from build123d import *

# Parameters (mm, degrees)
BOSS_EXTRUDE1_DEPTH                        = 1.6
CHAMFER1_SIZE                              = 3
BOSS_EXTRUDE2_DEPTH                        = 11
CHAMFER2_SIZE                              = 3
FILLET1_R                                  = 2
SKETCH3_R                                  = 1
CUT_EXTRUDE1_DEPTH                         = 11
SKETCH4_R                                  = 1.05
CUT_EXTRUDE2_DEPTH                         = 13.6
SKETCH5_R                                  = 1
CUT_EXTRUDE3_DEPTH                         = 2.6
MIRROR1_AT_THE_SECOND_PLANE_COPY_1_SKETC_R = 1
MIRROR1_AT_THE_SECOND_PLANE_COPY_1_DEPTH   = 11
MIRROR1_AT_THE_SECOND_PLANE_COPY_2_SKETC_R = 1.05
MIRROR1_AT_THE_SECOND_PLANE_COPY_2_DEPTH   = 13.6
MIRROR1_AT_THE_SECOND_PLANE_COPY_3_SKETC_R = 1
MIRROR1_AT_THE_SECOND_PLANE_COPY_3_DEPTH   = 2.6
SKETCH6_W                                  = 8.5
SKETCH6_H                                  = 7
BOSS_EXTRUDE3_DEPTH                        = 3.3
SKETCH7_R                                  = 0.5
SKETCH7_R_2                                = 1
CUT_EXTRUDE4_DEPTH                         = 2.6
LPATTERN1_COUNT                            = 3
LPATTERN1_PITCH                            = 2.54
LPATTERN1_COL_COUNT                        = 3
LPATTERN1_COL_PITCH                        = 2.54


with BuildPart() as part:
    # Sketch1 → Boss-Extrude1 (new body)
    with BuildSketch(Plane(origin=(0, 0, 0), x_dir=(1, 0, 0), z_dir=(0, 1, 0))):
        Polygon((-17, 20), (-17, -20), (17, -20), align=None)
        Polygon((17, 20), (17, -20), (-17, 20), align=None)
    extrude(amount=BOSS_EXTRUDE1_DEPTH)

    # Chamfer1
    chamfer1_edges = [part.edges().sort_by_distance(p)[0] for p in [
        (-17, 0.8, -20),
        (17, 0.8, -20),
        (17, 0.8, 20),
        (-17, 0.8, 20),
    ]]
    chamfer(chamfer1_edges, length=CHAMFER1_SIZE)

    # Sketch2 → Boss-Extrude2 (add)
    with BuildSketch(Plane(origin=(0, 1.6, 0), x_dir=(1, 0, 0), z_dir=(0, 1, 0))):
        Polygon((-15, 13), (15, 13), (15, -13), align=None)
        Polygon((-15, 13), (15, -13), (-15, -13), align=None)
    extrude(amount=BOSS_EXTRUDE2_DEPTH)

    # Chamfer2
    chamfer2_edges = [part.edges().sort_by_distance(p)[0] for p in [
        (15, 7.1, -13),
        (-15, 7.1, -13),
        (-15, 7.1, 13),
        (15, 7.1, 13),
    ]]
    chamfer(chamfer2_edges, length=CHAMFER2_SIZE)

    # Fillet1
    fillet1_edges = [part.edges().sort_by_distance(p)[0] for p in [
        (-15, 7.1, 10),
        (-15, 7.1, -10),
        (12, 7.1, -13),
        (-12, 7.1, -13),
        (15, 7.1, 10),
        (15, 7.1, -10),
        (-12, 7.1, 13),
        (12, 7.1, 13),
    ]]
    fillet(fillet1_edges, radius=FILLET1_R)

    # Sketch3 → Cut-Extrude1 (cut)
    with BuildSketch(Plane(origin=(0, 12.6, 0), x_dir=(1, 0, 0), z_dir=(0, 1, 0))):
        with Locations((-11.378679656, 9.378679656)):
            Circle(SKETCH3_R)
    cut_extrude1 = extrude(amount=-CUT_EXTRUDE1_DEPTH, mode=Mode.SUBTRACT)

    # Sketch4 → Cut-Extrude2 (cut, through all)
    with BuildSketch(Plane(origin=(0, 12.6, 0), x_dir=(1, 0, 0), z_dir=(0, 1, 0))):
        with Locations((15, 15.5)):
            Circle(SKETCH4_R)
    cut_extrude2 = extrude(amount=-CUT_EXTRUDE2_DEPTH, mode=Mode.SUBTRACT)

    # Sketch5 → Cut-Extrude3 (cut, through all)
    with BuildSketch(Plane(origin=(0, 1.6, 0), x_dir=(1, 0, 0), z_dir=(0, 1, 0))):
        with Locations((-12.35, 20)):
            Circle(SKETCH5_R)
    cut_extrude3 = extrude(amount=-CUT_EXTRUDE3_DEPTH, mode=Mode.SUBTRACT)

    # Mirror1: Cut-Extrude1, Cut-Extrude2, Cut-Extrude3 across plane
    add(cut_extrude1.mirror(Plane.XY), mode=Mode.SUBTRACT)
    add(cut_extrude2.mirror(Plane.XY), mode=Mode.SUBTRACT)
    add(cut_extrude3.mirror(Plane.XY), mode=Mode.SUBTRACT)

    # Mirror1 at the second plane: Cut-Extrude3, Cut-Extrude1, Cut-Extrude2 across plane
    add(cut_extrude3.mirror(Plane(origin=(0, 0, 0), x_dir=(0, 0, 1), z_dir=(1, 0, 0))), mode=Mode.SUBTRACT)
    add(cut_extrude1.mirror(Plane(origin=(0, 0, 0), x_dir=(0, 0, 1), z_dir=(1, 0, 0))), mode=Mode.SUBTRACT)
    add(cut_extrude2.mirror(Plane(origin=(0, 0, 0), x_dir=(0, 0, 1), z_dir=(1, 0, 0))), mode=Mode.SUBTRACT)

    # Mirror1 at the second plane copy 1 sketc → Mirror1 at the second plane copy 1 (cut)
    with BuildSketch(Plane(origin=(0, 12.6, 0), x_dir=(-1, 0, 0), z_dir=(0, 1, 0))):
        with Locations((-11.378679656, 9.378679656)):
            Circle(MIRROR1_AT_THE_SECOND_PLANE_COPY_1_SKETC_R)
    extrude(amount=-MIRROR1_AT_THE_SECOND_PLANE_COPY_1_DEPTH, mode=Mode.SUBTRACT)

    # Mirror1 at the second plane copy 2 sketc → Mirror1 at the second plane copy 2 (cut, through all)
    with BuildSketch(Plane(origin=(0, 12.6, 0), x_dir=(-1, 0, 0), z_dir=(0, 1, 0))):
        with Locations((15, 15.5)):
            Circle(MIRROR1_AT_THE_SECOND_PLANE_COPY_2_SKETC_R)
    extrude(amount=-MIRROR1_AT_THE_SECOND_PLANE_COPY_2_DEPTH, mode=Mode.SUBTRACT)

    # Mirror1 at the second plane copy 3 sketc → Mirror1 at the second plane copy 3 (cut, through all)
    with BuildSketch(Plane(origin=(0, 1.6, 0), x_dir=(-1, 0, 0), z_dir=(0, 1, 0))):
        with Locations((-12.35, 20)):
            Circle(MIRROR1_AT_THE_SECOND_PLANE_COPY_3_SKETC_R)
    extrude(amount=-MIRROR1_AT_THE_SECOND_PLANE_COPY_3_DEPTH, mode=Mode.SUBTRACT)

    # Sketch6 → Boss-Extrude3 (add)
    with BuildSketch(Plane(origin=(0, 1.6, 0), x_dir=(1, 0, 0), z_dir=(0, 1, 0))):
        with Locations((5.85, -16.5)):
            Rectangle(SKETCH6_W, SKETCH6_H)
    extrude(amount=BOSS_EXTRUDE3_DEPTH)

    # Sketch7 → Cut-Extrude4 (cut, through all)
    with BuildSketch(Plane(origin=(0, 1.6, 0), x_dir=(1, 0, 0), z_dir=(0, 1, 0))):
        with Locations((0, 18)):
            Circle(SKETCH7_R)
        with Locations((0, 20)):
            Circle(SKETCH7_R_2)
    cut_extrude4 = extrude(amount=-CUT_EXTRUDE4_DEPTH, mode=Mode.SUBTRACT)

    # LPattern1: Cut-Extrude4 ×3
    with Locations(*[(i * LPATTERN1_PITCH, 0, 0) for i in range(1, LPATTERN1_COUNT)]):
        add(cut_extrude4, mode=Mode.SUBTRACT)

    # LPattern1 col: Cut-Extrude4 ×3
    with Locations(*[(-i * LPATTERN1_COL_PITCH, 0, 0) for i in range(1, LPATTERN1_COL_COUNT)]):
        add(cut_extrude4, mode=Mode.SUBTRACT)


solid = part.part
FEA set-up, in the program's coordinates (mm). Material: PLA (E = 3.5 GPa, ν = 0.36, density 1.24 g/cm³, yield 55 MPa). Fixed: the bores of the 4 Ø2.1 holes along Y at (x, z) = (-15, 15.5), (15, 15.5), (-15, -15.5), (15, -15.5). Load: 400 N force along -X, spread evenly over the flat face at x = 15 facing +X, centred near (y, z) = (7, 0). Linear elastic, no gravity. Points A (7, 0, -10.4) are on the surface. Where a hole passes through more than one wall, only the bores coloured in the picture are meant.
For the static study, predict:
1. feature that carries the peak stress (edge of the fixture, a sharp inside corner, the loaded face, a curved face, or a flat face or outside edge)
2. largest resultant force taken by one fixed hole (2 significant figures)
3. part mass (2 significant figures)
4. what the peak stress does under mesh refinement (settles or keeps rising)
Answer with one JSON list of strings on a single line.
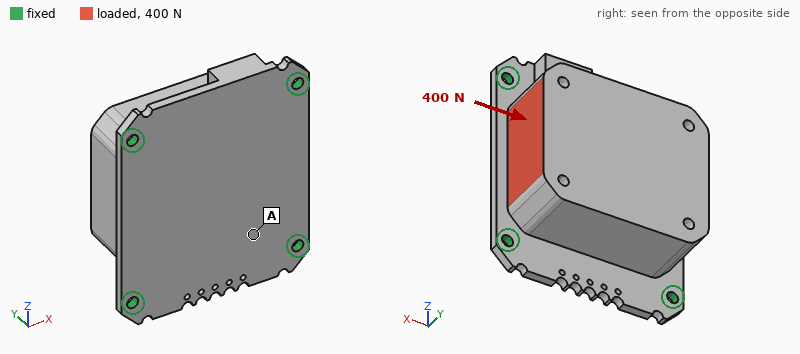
["edge of the fixture", "130 N", "13 g", "keeps rising"]
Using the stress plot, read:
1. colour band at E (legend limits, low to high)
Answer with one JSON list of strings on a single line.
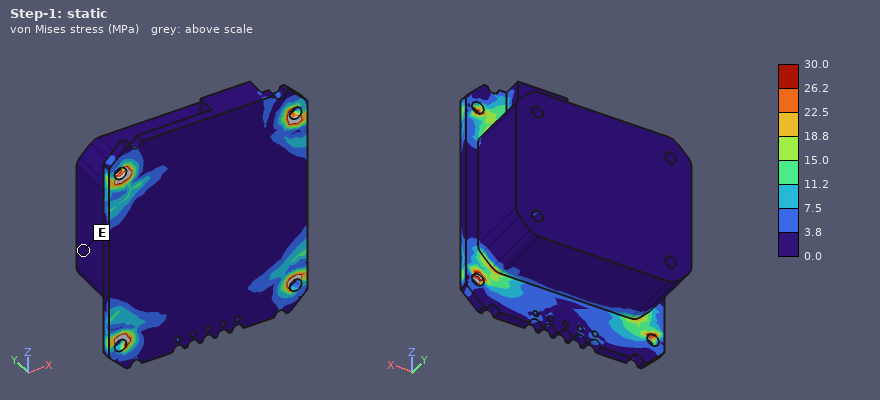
["0.0 to 3.8 MPa"]
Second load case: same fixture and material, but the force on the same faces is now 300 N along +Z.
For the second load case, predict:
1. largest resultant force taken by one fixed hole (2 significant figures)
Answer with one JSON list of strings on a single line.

["120 N"]
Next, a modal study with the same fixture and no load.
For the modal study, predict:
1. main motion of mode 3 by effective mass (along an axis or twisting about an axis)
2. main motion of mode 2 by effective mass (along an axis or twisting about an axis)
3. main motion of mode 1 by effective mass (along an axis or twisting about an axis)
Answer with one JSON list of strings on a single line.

["along Z", "along X", "along Y"]
